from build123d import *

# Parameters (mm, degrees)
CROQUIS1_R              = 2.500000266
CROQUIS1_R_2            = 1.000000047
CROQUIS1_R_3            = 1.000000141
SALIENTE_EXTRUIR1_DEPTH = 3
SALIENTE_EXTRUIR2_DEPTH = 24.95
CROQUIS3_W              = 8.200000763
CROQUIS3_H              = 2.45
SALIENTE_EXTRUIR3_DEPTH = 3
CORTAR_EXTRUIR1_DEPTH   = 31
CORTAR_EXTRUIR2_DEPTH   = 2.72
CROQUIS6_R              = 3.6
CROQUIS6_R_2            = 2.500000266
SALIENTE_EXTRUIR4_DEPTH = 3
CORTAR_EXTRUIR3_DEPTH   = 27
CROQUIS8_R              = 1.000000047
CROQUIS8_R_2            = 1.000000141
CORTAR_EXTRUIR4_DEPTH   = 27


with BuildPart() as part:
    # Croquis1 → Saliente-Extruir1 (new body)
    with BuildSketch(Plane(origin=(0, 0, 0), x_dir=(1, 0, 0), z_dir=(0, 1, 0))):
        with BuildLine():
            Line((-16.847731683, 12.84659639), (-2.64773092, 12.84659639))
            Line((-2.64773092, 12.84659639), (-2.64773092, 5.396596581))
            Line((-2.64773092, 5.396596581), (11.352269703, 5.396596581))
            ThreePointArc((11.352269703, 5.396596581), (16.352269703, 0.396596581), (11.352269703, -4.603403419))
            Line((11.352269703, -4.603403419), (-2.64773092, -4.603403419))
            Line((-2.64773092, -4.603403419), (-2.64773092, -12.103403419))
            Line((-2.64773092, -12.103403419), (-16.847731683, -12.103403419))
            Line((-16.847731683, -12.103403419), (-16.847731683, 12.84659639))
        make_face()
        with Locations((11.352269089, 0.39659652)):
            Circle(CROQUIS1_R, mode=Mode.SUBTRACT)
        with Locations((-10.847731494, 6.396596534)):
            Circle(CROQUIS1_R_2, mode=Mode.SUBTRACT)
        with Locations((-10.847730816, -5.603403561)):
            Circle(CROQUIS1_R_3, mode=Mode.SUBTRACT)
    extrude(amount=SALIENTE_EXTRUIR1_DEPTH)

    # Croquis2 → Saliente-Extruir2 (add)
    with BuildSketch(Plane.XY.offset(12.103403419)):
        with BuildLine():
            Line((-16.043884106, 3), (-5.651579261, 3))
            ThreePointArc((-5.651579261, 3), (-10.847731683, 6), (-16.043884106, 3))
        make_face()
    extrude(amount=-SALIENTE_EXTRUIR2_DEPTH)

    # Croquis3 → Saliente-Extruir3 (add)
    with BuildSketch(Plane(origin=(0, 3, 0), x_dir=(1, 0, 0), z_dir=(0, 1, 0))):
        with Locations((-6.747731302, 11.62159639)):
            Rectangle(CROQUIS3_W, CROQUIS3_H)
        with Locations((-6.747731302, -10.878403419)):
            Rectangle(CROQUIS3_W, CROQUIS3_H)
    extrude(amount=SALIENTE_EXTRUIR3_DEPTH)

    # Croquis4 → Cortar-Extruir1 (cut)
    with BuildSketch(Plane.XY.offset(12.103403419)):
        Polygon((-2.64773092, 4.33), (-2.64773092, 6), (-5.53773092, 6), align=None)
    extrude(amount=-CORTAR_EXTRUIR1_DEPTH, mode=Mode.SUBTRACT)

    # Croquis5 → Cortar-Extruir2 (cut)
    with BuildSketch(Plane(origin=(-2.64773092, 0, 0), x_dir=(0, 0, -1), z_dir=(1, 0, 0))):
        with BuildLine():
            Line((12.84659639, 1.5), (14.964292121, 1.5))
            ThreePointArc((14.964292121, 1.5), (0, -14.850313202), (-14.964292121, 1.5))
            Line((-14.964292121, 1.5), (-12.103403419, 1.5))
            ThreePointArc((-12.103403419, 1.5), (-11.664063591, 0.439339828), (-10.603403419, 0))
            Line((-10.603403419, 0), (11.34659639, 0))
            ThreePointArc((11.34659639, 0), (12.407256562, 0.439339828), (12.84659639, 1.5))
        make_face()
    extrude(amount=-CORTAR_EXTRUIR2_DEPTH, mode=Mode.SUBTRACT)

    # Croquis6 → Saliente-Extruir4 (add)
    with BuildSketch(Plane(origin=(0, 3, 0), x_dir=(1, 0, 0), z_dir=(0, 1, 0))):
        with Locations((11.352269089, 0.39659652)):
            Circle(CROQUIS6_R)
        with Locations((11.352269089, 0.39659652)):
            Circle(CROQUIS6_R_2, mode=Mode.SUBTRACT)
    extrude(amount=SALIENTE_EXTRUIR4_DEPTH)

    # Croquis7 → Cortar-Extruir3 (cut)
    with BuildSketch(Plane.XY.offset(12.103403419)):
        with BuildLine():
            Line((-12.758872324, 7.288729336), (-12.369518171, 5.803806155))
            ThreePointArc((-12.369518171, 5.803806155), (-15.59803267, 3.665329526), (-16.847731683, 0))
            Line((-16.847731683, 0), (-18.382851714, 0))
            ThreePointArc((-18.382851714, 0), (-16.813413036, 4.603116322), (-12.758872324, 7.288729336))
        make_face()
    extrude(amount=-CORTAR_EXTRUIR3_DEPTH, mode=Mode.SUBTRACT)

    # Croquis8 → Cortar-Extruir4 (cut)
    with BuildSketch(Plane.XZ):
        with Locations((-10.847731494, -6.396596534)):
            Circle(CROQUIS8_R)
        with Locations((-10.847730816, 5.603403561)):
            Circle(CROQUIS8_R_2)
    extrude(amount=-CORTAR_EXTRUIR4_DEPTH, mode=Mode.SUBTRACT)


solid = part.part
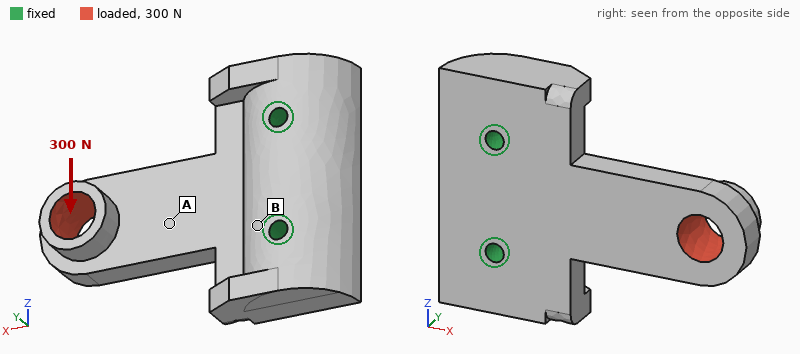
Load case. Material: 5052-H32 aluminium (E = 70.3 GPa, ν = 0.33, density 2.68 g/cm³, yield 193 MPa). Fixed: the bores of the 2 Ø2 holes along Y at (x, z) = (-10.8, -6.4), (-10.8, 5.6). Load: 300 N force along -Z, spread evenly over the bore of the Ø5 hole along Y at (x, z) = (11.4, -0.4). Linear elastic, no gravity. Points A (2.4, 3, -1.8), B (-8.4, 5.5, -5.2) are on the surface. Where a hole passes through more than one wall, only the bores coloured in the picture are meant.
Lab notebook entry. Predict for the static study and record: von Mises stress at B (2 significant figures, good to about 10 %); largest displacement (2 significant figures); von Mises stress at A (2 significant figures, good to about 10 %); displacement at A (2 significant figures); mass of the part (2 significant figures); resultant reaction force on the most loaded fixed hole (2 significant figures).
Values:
9.9 MPa
64 µm
55 MPa
14 µm
5.8 g
540 N
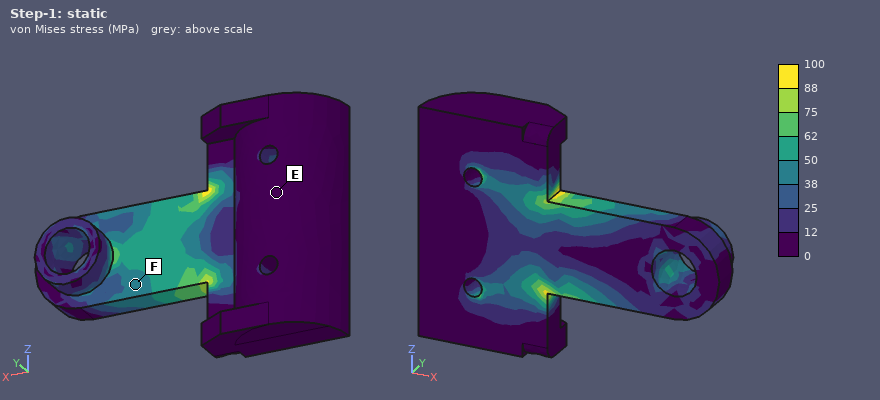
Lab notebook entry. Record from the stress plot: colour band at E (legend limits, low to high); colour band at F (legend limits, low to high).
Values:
0 to 12 MPa
38 to 50 MPa
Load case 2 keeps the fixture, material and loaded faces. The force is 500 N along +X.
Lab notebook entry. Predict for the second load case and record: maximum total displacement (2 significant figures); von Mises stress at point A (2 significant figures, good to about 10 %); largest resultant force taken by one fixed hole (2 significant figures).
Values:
0.11 mm
64 MPa
260 N
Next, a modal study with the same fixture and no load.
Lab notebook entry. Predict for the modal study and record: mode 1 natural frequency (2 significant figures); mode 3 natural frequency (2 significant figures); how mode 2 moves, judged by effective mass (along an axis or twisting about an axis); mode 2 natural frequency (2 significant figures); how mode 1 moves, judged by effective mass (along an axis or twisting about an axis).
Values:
5000 Hz
20 kHz
along Z
15 kHz
along Y
